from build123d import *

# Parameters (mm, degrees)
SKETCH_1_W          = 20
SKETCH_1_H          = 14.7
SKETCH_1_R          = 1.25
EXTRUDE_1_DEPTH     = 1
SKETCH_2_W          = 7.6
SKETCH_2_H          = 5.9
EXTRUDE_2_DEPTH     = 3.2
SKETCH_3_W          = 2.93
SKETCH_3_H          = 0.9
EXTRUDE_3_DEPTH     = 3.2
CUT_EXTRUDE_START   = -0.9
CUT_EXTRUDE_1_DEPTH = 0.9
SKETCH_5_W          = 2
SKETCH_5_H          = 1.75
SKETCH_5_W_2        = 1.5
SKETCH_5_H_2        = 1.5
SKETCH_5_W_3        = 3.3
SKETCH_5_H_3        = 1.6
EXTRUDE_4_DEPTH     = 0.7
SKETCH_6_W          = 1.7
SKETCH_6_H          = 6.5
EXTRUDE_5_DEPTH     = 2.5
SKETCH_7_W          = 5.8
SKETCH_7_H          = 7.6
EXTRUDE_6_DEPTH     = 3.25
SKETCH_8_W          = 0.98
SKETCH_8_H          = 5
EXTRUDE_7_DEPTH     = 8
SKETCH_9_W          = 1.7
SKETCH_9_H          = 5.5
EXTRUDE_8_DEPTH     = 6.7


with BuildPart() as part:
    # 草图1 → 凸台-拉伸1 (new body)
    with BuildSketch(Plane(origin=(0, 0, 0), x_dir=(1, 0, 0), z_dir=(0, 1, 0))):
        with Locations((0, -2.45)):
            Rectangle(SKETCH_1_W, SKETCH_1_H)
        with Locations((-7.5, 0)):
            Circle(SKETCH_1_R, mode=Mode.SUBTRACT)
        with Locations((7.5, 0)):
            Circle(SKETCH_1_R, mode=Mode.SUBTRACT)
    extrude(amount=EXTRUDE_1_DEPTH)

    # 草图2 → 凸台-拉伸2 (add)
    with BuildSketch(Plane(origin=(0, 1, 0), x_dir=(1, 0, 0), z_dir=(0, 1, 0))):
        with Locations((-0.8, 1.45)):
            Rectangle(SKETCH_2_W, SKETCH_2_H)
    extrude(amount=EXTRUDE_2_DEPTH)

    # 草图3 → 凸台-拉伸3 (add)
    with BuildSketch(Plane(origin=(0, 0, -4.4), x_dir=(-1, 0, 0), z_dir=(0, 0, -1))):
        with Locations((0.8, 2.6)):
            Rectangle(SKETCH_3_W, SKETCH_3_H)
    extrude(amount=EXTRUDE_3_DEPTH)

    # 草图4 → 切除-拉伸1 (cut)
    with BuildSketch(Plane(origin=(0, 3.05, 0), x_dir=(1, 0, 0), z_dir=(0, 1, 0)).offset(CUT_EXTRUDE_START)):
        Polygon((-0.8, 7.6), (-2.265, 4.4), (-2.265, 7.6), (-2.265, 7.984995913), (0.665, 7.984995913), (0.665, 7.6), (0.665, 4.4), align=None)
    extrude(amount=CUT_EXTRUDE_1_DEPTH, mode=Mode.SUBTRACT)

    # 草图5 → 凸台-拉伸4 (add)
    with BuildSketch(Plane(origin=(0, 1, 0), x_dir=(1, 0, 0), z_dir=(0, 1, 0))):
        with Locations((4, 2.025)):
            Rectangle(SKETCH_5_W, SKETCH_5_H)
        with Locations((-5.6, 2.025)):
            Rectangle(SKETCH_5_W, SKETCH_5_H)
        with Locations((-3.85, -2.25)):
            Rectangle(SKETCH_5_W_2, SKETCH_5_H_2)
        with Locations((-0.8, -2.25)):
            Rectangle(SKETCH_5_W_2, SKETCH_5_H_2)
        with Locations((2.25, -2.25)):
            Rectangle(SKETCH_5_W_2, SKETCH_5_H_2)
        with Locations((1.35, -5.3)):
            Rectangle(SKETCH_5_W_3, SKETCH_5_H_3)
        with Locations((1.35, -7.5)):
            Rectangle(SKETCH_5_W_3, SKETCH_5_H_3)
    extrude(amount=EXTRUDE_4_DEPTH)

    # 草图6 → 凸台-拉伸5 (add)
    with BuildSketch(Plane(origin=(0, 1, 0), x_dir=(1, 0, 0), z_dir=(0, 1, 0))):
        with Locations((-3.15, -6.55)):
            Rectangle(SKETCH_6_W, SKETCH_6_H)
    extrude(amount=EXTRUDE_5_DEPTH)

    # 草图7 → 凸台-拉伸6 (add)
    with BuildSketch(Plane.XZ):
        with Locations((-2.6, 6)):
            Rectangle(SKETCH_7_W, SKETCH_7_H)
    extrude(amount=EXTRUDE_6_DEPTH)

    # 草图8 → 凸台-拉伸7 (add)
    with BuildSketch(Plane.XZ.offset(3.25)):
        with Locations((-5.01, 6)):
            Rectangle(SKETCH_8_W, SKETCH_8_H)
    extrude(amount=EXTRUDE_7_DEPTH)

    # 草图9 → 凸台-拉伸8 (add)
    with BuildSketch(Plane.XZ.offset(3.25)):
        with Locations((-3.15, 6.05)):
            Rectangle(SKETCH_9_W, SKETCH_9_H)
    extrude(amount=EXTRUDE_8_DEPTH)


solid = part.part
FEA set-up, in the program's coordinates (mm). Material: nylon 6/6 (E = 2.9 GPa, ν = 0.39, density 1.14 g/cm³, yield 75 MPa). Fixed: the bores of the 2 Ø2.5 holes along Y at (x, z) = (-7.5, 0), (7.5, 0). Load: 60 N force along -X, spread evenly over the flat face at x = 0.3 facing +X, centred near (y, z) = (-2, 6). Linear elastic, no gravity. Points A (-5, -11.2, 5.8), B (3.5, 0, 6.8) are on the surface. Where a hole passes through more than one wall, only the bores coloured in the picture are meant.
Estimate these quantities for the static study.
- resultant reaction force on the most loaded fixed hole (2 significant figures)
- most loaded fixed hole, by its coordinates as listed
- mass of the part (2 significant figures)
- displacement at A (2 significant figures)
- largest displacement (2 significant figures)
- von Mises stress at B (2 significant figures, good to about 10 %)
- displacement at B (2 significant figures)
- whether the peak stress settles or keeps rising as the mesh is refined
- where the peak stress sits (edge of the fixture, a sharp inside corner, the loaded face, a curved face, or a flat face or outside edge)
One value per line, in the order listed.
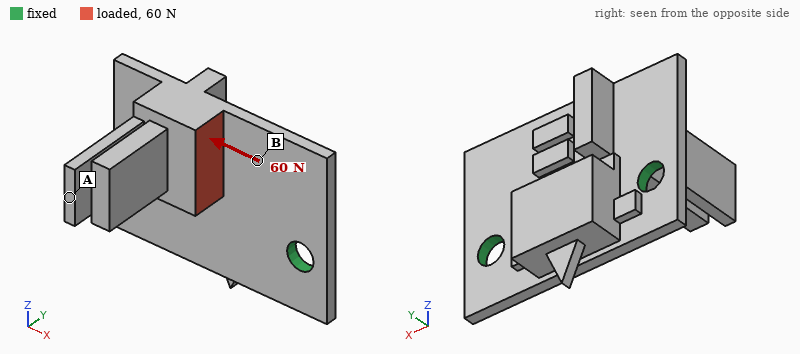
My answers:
45 N
(-7.5, 0)
0.82 g
0.16 mm
0.17 mm
8.8 MPa
0.075 mm
keeps rising
edge of the fixture
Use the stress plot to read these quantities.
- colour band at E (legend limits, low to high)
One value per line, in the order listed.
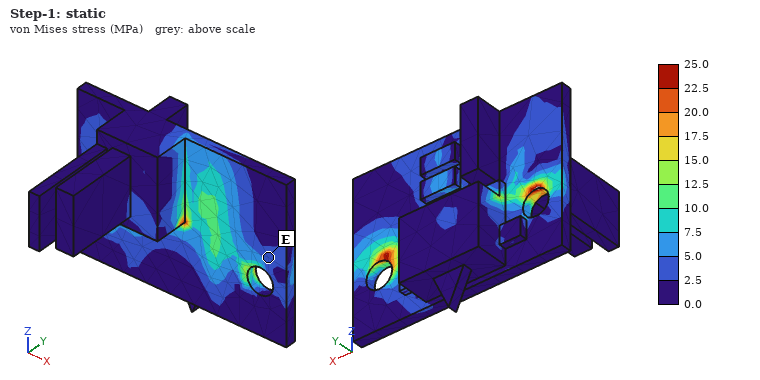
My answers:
2.5 to 5.0 MPa
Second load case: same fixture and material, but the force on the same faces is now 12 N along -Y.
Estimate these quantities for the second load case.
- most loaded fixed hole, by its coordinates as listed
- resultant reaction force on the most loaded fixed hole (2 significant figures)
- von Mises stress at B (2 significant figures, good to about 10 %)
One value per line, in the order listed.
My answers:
(7.5, 0)
7.1 N
4.9 MPa
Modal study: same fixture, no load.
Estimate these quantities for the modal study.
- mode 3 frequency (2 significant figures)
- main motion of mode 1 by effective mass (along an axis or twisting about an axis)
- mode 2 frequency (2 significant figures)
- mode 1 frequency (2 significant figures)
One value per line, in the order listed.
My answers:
5100 Hz
along Y
3300 Hz
1700 Hz
